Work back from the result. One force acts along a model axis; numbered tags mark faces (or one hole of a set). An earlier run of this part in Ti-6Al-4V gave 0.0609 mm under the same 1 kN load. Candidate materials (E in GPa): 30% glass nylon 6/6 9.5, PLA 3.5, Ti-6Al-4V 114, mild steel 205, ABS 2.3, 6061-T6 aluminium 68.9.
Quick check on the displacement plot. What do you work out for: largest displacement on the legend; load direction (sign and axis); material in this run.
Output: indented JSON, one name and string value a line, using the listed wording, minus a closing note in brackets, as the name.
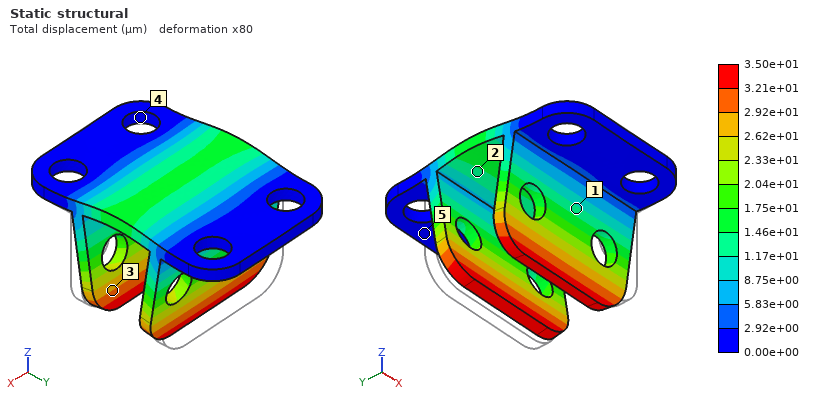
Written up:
{
  "largest displacement on the legend": "3.50e+01 µm",
  "load direction": "+Z",
  "material in this run": "mild steel"
}
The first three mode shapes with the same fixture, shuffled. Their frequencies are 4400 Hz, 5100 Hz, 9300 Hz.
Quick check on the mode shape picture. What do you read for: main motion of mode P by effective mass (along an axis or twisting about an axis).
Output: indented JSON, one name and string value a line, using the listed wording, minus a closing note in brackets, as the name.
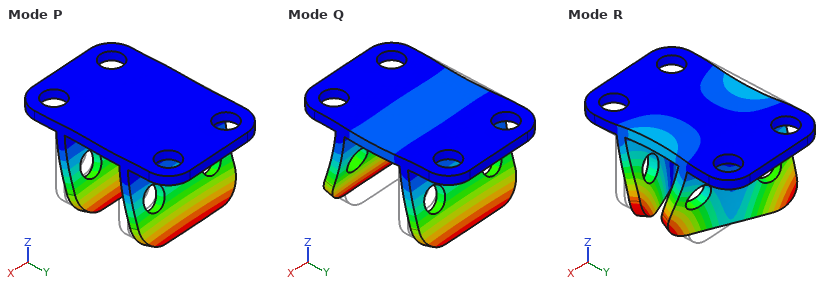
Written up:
{
  "main motion of mode P by effective mass": "along Y"
}
